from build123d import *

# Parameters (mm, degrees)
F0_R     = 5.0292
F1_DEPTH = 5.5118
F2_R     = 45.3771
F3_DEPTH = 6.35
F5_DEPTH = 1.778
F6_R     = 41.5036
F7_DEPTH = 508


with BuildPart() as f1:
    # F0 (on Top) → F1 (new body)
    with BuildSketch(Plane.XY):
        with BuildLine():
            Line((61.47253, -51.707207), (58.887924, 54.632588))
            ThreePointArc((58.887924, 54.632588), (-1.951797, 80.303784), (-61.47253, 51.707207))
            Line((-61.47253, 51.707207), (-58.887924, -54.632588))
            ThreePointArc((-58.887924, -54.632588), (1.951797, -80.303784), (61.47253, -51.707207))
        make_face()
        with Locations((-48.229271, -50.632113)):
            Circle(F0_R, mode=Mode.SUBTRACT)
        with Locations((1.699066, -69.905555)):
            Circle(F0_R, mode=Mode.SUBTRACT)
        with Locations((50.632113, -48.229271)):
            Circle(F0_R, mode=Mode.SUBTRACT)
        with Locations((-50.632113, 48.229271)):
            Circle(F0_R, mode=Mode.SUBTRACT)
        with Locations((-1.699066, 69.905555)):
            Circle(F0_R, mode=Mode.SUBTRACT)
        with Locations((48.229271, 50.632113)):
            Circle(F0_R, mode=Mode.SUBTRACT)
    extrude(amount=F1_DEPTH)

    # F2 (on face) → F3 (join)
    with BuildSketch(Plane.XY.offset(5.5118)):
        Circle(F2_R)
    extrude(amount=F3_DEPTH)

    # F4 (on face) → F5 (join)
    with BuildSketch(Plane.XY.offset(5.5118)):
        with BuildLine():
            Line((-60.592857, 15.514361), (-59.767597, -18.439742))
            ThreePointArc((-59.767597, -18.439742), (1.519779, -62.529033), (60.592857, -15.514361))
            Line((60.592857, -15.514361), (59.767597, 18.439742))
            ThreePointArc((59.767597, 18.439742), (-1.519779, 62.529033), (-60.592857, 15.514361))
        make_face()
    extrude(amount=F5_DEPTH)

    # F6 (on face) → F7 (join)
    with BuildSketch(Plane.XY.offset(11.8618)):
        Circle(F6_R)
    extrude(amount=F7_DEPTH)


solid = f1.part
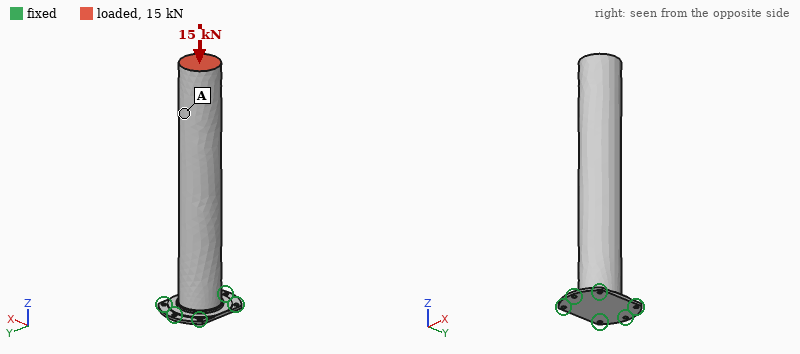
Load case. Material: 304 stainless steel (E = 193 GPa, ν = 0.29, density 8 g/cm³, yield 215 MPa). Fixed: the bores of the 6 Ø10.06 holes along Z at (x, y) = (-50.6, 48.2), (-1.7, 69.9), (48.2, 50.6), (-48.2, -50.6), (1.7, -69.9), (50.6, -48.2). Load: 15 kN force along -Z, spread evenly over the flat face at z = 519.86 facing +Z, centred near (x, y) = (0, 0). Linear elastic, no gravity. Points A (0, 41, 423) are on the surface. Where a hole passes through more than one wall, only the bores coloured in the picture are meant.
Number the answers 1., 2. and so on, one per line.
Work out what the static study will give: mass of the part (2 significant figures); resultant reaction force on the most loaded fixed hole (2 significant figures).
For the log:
1. 23 kg
2. 3.6 kN
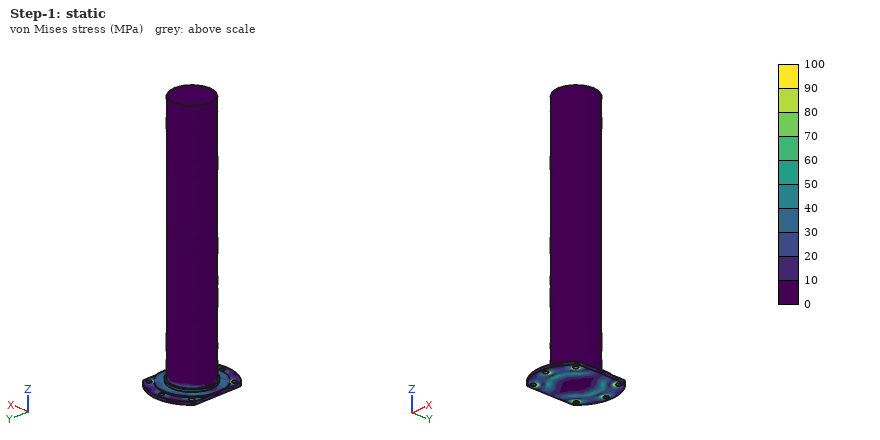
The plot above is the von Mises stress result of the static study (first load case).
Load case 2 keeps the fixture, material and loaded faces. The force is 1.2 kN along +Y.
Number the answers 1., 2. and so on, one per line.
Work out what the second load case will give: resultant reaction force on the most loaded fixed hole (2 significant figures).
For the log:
1. 2.7 kN
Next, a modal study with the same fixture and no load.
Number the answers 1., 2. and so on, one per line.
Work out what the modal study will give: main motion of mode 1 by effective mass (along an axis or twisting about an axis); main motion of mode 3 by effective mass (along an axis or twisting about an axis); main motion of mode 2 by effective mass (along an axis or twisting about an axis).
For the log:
1. along X
2. along Z
3. along Y
